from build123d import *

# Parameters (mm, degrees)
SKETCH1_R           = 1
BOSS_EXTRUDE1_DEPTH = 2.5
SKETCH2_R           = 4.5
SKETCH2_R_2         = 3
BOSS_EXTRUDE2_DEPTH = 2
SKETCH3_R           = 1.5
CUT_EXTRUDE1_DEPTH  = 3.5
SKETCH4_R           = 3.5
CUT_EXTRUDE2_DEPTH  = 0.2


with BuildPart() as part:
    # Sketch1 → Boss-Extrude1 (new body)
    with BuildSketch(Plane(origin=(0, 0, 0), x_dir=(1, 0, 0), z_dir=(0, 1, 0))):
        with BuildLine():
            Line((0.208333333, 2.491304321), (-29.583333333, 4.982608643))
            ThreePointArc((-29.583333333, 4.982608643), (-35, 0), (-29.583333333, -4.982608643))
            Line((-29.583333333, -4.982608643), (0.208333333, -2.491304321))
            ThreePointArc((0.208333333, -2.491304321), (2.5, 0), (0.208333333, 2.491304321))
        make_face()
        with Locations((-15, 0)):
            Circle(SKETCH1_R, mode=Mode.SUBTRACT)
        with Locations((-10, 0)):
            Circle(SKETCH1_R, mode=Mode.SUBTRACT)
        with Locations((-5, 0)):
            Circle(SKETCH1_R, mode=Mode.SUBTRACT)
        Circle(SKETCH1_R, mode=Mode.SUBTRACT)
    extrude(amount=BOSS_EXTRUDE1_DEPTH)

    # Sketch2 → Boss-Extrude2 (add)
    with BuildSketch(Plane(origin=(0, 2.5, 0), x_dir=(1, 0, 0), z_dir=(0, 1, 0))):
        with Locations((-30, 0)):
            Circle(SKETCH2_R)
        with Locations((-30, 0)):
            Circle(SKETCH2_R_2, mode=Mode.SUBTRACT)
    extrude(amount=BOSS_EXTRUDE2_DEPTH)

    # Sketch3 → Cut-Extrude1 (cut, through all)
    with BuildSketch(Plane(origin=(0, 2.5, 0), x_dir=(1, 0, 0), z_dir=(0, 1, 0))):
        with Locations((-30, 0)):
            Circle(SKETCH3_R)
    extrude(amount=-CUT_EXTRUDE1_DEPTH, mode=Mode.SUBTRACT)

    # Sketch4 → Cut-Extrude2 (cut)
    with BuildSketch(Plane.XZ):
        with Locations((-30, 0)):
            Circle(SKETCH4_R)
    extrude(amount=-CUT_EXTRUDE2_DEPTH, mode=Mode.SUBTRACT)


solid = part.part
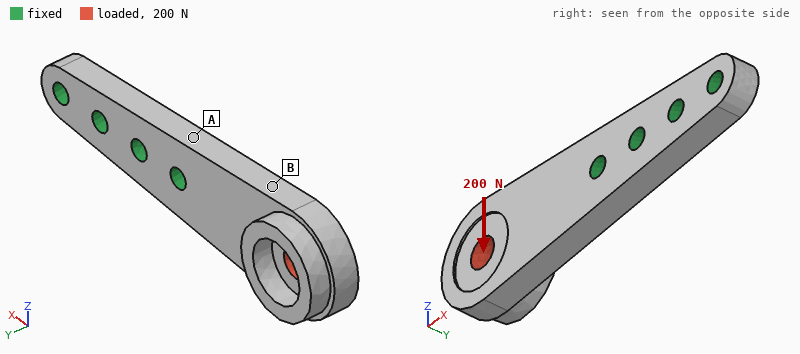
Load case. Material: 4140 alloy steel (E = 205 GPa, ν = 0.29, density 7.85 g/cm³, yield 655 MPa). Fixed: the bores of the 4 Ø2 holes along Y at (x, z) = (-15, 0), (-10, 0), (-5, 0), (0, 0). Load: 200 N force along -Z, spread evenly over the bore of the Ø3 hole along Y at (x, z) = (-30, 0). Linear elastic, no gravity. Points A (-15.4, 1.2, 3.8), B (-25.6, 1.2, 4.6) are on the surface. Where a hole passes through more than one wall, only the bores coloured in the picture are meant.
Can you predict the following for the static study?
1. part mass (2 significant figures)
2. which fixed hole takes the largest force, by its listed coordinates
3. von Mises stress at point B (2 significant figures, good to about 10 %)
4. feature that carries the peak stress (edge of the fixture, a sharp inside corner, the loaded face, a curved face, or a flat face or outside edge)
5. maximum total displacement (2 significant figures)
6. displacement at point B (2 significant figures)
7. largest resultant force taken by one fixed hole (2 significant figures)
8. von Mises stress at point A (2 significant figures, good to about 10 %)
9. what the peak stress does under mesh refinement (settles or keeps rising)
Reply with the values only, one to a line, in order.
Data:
5.5 g
(-15, 0)
24 MPa
edge of the fixture
26 µm
13 µm
490 N
110 MPa
keeps rising
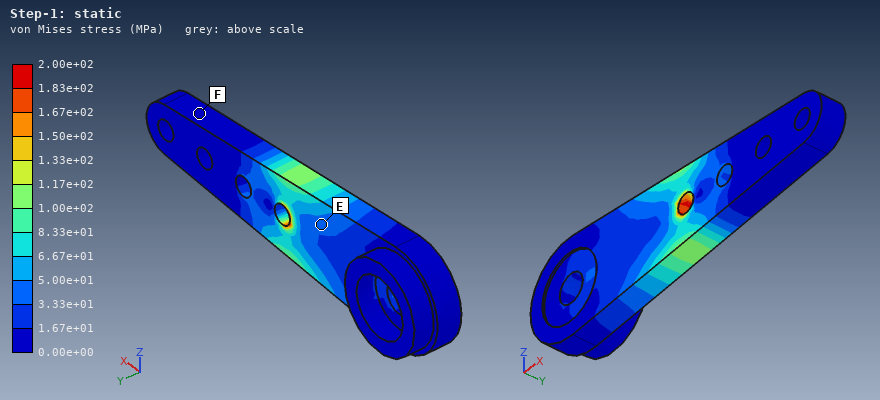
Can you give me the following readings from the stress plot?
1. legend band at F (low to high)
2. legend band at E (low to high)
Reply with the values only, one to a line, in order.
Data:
0.00e+00 to 1.67e+01 MPa
3.33e+01 to 5.00e+01 MPa
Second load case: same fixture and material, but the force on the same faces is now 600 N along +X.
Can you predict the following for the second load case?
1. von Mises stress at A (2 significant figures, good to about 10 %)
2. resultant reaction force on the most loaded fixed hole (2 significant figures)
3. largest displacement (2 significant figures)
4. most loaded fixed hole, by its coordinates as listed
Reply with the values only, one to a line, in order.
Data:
19 MPa
500 N
4.7 µm
(-15, 0)
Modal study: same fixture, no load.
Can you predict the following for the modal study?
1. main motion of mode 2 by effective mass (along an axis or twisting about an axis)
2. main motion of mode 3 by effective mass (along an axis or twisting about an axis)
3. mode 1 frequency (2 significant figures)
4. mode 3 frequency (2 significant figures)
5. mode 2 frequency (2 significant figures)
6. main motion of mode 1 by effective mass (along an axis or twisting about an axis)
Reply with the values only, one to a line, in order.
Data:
along Z
twisting about X
4700 Hz
17 kHz
11 kHz
along Y
